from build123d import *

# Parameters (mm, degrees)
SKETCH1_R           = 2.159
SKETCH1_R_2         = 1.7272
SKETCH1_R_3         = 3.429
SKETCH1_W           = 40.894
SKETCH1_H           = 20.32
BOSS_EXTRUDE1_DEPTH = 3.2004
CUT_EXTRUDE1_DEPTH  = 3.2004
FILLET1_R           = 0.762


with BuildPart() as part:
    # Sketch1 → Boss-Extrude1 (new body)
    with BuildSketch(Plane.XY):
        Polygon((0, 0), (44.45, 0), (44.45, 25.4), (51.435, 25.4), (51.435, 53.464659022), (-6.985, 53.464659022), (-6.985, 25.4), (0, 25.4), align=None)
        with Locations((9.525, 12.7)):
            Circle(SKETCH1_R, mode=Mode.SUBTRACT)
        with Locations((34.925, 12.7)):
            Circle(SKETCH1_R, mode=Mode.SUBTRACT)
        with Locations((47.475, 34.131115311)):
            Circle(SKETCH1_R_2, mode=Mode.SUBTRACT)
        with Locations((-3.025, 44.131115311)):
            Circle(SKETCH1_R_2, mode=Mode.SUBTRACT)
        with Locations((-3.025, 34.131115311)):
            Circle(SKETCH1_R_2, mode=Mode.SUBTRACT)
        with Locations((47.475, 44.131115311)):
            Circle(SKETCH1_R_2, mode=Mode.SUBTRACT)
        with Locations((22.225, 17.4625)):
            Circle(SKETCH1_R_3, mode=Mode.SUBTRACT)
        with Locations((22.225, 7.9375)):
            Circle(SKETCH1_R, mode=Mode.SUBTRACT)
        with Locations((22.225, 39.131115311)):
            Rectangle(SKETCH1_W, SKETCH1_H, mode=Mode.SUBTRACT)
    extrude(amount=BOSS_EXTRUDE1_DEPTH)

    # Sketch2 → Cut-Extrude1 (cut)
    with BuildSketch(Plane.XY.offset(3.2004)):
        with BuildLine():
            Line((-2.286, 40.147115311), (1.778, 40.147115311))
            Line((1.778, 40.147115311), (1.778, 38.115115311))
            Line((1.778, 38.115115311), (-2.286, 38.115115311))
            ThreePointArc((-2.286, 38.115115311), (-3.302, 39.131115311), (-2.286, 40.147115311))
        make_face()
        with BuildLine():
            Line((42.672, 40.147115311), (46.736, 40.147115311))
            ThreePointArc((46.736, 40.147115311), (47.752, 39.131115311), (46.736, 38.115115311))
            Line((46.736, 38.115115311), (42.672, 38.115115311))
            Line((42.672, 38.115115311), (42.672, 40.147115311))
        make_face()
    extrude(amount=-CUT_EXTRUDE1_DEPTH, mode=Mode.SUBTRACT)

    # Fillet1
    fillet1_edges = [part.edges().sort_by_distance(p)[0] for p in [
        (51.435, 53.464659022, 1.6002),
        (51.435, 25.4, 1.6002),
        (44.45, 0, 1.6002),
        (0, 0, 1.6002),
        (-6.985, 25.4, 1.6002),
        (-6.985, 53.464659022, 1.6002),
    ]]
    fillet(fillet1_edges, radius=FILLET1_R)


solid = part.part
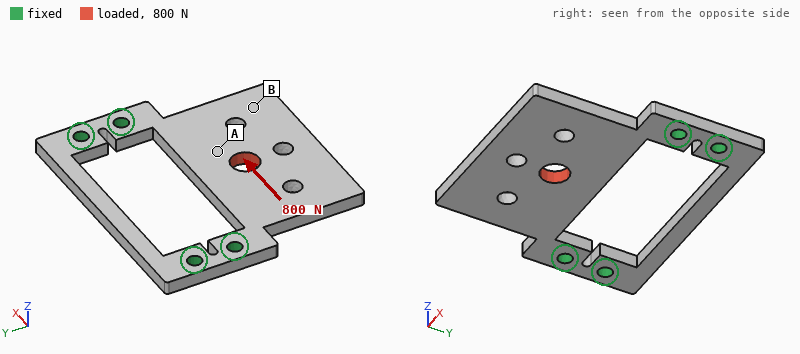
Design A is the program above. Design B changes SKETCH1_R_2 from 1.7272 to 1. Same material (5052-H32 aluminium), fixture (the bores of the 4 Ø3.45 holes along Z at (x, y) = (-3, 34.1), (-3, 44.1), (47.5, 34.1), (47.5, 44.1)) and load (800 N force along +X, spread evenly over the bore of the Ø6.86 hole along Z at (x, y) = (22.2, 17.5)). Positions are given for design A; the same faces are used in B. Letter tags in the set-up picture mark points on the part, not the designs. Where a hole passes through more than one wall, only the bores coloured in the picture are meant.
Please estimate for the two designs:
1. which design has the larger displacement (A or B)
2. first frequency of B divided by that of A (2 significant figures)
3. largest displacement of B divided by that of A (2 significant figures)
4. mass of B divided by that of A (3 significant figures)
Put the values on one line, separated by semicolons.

B; 0.95; 1.2; 1.01
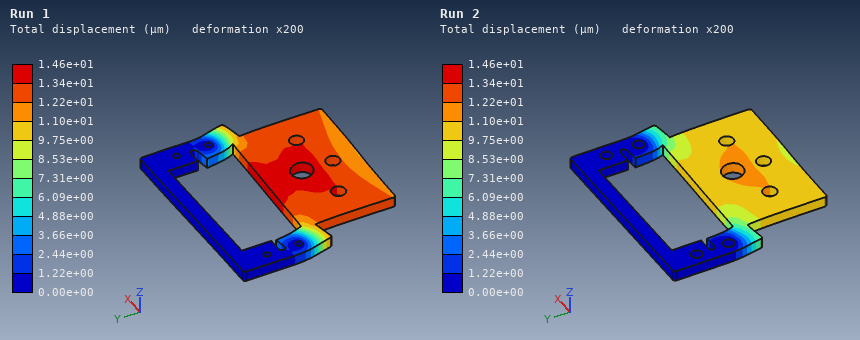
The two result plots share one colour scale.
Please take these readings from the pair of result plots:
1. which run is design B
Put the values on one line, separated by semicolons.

Run 1
